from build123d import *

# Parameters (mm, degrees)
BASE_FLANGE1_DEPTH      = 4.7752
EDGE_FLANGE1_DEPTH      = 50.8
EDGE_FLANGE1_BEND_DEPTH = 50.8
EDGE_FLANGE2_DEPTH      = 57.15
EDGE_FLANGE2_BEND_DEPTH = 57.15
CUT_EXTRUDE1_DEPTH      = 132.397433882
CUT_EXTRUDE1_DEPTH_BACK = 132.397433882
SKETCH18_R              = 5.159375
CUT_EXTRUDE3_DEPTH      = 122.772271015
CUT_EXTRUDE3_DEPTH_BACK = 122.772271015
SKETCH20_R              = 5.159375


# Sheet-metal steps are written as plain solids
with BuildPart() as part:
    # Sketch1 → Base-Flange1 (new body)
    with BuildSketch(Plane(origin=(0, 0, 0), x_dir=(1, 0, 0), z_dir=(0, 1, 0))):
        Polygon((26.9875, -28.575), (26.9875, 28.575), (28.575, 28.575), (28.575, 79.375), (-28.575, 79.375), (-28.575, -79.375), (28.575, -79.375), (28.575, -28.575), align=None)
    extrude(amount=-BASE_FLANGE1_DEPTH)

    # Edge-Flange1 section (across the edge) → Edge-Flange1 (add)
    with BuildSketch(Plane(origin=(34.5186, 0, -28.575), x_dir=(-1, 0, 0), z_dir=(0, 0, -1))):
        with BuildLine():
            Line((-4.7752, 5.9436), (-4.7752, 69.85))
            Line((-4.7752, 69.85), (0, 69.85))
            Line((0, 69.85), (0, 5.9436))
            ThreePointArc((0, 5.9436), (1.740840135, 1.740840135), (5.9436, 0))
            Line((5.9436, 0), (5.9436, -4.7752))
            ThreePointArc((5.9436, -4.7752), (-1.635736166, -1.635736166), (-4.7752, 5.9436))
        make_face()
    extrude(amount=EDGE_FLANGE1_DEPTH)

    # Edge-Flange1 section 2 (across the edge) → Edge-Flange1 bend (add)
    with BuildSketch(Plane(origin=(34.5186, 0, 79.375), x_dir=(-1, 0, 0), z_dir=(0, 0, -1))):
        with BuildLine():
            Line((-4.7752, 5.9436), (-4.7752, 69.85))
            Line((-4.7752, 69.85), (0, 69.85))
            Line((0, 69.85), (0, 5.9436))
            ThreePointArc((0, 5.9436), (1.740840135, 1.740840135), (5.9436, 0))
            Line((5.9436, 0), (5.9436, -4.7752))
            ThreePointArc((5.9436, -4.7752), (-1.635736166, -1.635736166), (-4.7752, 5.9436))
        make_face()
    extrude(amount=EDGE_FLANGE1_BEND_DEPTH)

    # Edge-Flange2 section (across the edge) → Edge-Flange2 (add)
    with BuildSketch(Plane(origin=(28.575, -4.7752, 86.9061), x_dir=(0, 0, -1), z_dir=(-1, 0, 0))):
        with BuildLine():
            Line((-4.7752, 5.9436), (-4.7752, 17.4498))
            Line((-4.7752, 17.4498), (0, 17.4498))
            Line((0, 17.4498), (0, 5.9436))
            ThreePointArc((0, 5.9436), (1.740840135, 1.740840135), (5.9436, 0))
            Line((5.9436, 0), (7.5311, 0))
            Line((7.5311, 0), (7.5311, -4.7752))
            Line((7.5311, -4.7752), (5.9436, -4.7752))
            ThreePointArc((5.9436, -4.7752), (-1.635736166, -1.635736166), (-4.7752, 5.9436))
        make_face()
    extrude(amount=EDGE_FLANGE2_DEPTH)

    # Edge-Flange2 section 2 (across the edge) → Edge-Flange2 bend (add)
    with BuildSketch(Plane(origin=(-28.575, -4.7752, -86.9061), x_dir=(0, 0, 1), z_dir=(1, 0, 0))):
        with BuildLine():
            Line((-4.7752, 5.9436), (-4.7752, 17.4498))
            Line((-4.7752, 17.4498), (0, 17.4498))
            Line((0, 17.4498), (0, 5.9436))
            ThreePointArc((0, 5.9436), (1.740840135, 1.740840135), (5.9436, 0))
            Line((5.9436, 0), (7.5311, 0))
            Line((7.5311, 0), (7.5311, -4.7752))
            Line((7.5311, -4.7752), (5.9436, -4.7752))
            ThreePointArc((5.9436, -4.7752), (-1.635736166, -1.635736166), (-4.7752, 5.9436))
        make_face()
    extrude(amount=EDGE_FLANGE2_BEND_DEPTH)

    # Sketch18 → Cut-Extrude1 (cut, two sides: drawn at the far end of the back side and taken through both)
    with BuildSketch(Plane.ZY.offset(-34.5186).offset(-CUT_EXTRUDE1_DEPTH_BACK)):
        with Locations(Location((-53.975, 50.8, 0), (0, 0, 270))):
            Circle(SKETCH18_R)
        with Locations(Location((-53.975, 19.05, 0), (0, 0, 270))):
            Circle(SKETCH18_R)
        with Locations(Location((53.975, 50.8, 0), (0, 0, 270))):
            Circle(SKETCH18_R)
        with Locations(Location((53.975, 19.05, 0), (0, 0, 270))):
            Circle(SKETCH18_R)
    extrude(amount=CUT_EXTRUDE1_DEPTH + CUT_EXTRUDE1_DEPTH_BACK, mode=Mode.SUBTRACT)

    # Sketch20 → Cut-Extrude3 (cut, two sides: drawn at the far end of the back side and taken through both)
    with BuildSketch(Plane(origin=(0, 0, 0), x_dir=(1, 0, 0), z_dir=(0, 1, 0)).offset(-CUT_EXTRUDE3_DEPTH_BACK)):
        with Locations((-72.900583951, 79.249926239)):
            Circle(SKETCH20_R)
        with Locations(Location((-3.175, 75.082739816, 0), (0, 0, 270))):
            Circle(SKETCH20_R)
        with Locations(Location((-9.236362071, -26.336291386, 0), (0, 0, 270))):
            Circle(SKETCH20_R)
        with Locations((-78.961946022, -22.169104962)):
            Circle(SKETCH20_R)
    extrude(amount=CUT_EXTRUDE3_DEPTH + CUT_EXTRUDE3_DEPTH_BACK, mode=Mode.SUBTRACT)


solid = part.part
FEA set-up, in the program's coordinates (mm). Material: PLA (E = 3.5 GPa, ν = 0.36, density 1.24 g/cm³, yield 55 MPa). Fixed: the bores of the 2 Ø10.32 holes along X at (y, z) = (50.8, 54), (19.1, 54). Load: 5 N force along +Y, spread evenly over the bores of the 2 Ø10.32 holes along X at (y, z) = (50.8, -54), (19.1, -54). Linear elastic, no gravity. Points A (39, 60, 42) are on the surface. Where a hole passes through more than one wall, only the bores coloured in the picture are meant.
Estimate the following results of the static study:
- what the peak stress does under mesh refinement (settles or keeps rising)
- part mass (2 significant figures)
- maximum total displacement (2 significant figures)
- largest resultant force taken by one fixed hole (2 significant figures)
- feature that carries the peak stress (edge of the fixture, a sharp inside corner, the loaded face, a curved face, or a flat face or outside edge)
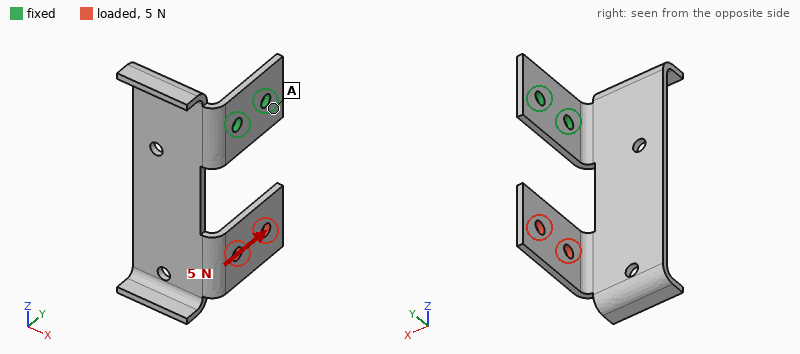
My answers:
keeps rising
110 g
2.3 mm
12 N
a sharp inside corner
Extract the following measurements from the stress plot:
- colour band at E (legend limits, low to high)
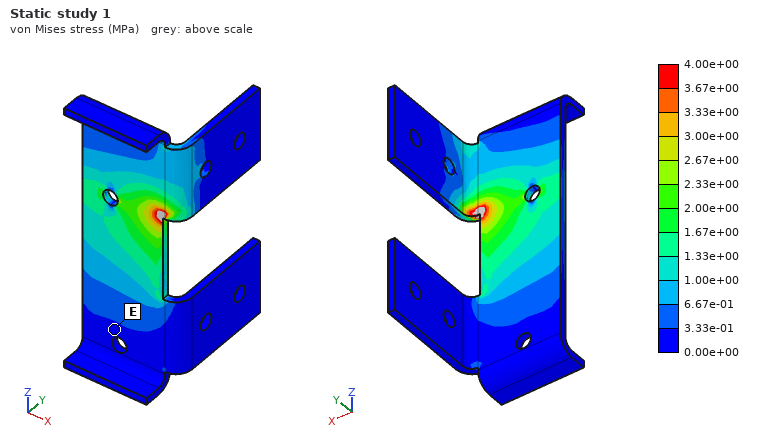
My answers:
0.00e+00 to 3.33e-01 MPa
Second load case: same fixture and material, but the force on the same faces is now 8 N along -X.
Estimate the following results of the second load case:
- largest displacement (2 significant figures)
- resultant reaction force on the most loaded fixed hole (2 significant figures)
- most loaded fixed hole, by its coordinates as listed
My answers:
2.3 mm
7.2 N
(19.1, 54)
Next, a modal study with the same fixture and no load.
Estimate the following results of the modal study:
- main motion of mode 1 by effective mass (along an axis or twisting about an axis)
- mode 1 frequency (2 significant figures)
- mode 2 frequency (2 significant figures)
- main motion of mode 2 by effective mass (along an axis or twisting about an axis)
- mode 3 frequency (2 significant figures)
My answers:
along Y
37 Hz
67 Hz
along X
87 Hz
